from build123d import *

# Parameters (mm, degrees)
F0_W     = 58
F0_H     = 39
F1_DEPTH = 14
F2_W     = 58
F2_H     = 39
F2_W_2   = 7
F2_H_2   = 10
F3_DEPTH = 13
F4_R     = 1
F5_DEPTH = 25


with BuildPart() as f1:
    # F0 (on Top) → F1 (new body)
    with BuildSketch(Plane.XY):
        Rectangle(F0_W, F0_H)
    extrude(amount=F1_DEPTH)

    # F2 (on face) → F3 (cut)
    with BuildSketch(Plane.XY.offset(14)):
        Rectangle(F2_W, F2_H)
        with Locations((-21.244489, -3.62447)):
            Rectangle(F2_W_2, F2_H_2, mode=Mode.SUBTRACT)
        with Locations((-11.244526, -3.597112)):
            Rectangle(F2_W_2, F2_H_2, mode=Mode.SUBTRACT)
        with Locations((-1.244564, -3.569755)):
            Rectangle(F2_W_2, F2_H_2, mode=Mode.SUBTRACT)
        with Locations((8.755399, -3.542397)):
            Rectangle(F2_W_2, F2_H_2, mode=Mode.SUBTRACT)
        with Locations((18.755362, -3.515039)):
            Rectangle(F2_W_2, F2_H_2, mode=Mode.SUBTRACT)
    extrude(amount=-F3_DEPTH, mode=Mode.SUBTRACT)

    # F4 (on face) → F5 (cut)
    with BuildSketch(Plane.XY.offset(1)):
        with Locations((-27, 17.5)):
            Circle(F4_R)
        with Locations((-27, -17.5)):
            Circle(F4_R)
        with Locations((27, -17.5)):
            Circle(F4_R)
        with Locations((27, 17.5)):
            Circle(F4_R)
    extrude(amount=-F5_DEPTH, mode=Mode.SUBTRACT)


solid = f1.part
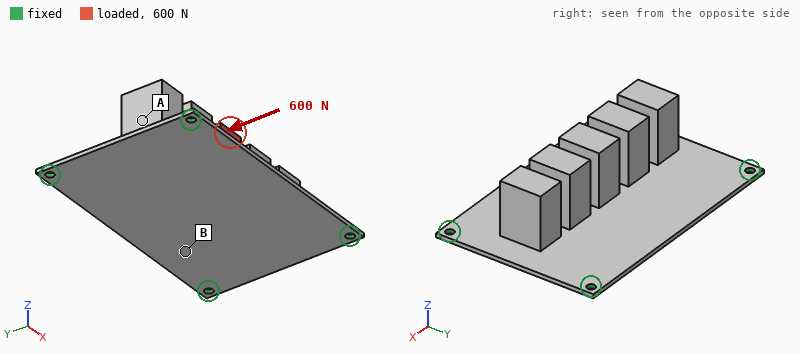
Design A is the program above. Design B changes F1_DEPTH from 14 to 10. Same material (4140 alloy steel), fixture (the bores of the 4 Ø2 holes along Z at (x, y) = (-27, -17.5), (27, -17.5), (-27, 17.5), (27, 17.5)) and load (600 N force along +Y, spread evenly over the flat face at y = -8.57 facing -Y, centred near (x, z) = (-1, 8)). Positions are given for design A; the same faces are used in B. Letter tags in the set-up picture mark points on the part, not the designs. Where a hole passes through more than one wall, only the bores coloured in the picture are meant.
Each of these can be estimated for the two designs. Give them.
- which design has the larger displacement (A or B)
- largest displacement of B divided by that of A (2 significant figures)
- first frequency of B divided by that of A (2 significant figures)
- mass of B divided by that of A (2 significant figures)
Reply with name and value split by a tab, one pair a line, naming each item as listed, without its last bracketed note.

which design has the larger displacement	A
largest displacement of B divided by that of A	0.60
first frequency of B divided by that of A	1.2
mass of B divided by that of A	0.79
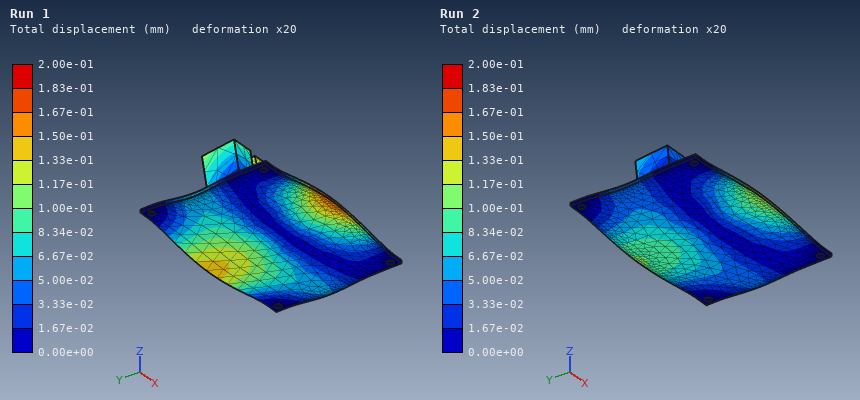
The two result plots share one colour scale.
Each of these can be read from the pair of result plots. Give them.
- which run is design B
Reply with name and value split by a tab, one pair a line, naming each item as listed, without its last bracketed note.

which run is design B	Run 2
